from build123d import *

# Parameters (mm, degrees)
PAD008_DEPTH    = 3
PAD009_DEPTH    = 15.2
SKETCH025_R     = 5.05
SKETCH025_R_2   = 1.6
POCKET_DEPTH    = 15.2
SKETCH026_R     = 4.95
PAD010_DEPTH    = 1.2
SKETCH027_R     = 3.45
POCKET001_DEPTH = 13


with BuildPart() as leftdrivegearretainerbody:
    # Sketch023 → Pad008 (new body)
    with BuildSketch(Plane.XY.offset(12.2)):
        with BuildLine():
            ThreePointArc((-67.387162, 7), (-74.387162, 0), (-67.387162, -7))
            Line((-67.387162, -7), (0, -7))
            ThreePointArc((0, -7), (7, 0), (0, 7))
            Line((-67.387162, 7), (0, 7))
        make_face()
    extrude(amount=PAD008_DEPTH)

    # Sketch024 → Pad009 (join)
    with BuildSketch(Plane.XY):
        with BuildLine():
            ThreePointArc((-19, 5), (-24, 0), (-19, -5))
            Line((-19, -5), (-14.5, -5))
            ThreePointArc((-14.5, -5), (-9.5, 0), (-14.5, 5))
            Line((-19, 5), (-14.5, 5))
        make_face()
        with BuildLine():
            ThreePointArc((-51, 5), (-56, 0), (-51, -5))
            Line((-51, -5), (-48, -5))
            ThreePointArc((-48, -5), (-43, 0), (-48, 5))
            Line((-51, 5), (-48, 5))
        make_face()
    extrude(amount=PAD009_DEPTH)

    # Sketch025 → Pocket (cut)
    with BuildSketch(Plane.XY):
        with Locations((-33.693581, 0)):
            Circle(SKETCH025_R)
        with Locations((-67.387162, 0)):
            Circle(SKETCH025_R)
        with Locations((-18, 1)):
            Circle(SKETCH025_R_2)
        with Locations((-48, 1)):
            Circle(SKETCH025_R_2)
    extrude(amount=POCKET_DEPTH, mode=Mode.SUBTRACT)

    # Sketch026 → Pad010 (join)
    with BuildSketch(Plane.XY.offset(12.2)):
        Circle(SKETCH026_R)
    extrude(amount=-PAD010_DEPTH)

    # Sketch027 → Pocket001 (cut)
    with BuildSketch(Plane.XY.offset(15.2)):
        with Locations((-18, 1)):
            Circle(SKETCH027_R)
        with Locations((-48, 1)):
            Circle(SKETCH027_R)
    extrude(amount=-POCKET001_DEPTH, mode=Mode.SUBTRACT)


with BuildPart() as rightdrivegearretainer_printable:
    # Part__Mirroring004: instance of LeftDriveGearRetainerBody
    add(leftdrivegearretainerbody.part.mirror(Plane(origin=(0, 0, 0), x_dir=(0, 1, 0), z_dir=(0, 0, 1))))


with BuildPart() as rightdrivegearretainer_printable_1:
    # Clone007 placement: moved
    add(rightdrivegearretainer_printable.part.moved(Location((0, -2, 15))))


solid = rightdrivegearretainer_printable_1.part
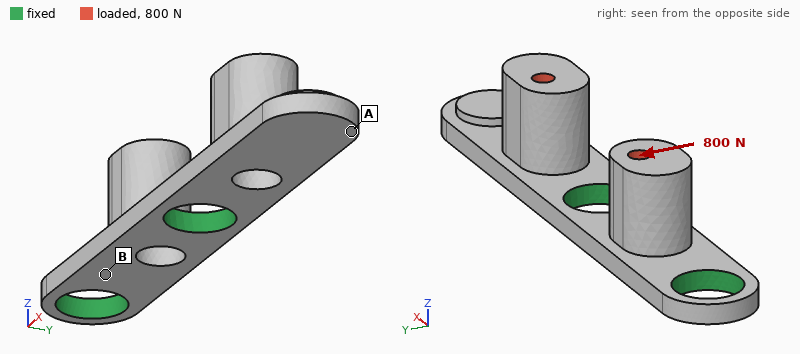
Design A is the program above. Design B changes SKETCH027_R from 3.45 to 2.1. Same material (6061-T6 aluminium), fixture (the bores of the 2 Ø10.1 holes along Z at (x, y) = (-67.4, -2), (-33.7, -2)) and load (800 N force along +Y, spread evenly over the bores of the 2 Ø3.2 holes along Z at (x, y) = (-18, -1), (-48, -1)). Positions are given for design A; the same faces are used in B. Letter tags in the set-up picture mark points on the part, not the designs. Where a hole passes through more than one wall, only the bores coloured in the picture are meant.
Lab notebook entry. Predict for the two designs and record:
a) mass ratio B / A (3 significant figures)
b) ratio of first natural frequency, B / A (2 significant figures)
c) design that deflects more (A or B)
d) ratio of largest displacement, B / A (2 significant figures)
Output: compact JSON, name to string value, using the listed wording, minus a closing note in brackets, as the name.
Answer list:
{"mass ratio B / A": "1.13", "ratio of first natural frequency, B / A": "1.0", "design that deflects more": "A", "ratio of largest displacement, B / A": "0.89"}
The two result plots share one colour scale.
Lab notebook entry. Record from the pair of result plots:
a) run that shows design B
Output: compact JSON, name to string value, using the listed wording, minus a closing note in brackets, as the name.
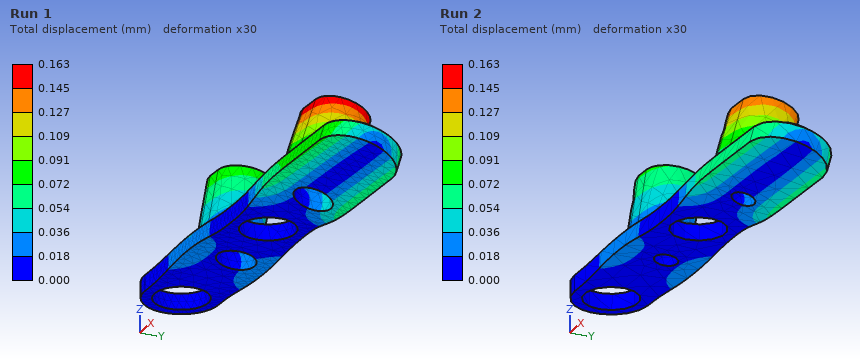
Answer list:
{"run that shows design B": "Run 2"}
